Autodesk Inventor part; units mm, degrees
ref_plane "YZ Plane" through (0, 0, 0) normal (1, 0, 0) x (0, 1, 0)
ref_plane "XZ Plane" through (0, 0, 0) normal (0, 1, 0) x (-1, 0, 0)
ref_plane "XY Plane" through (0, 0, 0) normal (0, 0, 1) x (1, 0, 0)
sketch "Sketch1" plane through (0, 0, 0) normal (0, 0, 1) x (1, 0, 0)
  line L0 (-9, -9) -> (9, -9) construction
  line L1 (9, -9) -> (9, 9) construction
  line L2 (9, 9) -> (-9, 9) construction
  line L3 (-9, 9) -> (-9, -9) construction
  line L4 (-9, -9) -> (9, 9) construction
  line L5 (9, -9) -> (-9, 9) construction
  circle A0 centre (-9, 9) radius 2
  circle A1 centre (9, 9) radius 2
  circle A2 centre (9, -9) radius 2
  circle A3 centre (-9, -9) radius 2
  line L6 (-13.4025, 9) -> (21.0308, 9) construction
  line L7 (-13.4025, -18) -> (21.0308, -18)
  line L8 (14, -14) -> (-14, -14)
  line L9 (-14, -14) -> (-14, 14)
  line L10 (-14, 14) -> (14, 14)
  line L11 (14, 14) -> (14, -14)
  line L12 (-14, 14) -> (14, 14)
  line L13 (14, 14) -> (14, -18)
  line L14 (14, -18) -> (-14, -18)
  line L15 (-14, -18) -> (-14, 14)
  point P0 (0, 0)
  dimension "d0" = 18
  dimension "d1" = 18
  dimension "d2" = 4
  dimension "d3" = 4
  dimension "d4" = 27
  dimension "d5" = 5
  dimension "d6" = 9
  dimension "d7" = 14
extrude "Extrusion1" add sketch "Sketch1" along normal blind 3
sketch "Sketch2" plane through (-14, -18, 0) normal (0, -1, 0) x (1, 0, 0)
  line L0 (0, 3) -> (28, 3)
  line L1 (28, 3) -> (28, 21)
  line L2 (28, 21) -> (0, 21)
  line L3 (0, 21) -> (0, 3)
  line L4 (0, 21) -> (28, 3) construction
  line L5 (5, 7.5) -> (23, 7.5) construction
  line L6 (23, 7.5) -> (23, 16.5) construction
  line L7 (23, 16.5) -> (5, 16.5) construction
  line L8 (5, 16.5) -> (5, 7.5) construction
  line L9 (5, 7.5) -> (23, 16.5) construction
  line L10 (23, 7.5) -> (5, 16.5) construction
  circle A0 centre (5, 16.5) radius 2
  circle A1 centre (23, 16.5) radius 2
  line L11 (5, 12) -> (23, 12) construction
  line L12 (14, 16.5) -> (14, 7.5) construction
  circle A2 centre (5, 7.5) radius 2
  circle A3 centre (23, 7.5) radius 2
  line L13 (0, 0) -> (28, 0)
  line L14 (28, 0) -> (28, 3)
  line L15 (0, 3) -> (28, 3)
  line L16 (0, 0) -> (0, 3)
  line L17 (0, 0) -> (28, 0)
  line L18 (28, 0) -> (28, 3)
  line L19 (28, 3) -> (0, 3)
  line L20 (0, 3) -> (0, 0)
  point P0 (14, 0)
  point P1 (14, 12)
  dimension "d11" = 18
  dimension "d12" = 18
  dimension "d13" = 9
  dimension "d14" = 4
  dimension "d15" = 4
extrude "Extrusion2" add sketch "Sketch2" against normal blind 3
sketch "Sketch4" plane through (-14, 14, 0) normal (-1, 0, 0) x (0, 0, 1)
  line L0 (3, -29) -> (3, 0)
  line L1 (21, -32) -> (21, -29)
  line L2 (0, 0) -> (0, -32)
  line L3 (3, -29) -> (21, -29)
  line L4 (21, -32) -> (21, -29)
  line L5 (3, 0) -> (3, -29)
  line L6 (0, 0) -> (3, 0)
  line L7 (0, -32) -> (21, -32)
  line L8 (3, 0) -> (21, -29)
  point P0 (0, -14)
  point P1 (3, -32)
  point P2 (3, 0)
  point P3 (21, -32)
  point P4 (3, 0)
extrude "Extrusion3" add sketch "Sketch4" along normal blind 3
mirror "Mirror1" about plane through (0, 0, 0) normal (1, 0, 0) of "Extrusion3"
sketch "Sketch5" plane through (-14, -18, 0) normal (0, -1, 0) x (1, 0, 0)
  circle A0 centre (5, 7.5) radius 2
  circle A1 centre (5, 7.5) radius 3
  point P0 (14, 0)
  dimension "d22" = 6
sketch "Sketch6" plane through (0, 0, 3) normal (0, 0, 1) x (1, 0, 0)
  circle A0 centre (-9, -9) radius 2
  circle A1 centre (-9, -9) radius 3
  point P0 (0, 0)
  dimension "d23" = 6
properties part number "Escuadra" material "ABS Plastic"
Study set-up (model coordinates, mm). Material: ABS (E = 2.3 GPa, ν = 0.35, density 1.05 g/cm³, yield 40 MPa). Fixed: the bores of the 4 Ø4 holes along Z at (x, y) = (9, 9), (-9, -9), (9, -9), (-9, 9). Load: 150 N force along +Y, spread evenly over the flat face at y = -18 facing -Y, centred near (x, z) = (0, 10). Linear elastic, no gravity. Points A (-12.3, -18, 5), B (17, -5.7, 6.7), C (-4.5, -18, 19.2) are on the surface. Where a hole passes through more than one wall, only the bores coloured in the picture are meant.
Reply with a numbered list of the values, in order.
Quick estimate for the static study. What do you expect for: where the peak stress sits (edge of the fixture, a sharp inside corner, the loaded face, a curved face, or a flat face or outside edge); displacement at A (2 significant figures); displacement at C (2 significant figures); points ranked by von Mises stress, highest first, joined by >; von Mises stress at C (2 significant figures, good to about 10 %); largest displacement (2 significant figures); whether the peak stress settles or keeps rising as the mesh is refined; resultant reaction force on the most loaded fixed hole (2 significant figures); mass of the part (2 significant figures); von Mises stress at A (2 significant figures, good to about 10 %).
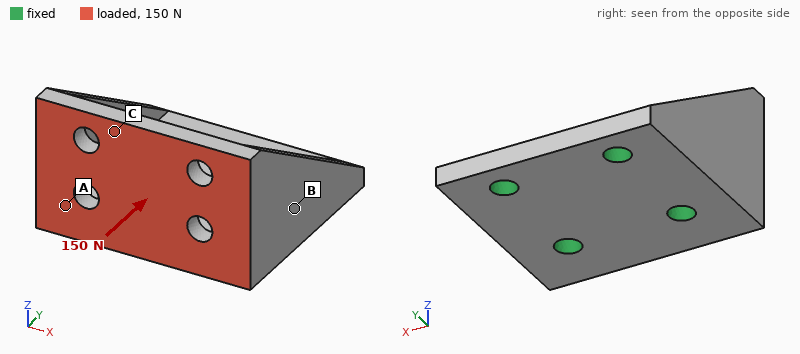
1. edge of the fixture
2. 0.052 mm
3. 0.24 mm
4. C > A > B
5. 6.2 MPa
6. 0.29 mm
7. keeps rising
8. 60 N
9. 6.7 g
10. 3.4 MPa
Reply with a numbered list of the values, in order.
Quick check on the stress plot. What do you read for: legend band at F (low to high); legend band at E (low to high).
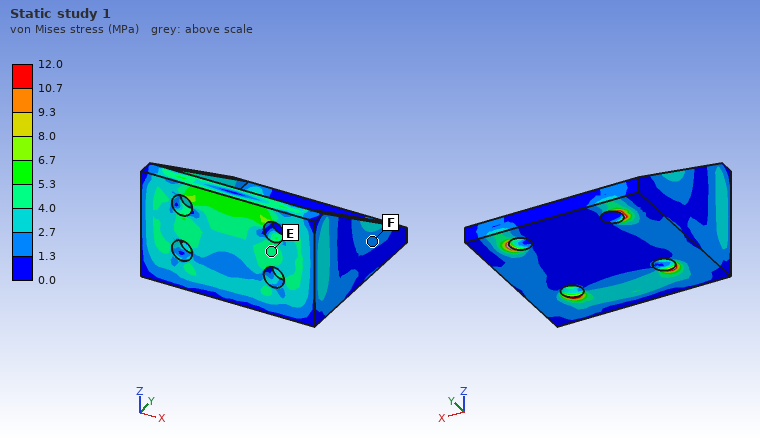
1. 1.3 to 2.7 MPa
2. 4.0 to 5.3 MPa
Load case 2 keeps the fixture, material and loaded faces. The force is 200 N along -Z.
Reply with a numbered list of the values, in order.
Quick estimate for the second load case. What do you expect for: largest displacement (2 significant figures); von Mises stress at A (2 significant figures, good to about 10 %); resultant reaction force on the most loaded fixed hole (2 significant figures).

1. 0.22 mm
2. 2.7 MPa
3. 130 N
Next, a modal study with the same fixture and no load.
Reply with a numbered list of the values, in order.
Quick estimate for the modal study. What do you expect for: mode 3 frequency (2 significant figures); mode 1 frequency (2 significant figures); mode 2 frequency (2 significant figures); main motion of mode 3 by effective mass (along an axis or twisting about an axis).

1. 5000 Hz
2. 3000 Hz
3. 3100 Hz
4. along Z
